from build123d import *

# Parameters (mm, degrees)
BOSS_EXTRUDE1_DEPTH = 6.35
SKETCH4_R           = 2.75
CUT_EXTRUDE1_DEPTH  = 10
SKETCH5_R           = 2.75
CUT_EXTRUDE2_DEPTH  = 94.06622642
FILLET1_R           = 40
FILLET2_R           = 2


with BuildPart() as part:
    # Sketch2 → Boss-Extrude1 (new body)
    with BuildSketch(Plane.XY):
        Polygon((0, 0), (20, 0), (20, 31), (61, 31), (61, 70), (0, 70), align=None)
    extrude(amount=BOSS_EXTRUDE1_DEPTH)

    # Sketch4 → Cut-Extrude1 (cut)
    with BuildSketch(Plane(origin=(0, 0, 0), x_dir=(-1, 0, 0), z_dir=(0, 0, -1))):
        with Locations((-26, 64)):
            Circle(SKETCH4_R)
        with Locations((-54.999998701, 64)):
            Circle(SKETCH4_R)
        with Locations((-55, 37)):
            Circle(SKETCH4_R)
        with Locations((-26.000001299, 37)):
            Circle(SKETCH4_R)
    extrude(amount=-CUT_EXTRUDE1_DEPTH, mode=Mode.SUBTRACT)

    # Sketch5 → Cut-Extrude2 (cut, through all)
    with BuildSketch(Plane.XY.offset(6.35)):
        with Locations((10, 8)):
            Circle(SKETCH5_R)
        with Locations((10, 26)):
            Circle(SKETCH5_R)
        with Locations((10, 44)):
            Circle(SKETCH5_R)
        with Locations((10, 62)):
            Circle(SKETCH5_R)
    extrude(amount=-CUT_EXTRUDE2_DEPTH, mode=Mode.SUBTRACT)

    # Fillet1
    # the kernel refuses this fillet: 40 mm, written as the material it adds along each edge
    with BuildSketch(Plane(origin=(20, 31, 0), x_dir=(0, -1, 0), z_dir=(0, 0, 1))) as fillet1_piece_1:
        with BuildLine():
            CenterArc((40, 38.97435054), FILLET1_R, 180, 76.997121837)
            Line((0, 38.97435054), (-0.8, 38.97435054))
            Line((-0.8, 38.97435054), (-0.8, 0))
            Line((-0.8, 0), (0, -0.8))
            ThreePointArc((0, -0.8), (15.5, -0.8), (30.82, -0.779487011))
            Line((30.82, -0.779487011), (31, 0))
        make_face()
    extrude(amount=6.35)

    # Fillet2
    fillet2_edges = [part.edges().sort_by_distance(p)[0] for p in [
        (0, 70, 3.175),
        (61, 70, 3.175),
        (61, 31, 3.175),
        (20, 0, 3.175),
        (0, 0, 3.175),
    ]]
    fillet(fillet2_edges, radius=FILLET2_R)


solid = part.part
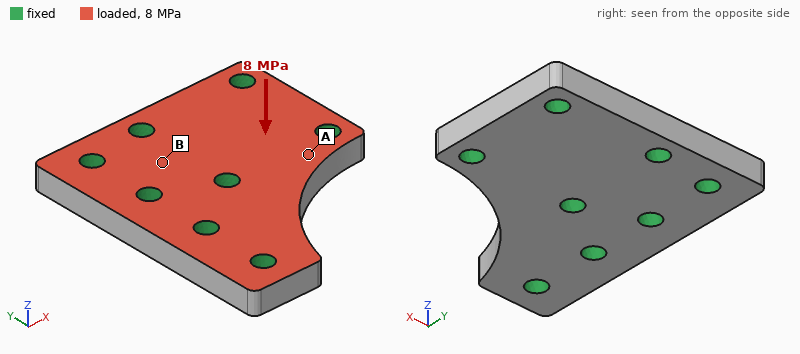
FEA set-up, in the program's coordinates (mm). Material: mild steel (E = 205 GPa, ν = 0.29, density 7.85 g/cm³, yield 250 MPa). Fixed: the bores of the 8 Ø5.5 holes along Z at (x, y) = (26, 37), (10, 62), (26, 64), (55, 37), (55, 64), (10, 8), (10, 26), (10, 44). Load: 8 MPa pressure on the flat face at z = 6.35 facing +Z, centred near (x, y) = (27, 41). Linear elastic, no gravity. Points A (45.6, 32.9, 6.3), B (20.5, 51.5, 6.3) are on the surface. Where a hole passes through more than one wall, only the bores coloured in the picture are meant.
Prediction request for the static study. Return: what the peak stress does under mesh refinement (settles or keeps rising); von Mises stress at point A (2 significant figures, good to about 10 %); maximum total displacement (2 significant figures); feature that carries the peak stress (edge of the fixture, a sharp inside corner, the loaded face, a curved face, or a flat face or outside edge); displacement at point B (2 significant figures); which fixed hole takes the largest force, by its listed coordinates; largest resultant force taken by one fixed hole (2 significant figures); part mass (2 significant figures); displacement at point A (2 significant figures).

keeps rising
38 MPa
12 µm
edge of the fixture
2.4 µm
(26, 37)
4.7 kN
160 g
5.1 µm
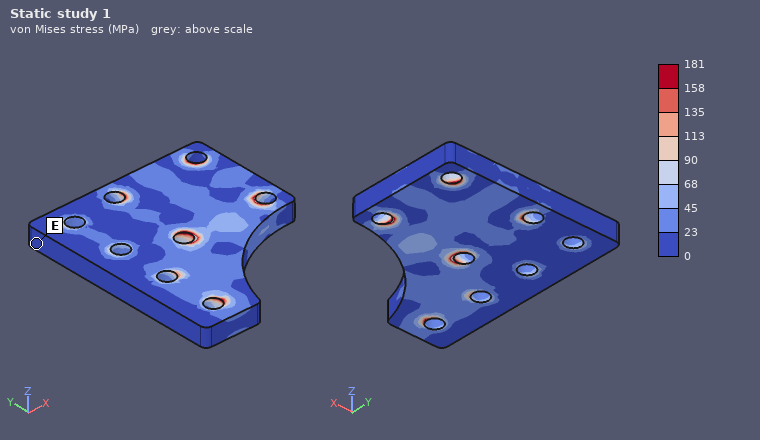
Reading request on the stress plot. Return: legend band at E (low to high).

0 to 23 MPa
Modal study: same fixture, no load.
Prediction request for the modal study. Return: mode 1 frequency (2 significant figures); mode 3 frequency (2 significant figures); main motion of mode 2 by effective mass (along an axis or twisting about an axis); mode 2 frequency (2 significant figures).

24 kHz
36 kHz
along Z
29 kHz
